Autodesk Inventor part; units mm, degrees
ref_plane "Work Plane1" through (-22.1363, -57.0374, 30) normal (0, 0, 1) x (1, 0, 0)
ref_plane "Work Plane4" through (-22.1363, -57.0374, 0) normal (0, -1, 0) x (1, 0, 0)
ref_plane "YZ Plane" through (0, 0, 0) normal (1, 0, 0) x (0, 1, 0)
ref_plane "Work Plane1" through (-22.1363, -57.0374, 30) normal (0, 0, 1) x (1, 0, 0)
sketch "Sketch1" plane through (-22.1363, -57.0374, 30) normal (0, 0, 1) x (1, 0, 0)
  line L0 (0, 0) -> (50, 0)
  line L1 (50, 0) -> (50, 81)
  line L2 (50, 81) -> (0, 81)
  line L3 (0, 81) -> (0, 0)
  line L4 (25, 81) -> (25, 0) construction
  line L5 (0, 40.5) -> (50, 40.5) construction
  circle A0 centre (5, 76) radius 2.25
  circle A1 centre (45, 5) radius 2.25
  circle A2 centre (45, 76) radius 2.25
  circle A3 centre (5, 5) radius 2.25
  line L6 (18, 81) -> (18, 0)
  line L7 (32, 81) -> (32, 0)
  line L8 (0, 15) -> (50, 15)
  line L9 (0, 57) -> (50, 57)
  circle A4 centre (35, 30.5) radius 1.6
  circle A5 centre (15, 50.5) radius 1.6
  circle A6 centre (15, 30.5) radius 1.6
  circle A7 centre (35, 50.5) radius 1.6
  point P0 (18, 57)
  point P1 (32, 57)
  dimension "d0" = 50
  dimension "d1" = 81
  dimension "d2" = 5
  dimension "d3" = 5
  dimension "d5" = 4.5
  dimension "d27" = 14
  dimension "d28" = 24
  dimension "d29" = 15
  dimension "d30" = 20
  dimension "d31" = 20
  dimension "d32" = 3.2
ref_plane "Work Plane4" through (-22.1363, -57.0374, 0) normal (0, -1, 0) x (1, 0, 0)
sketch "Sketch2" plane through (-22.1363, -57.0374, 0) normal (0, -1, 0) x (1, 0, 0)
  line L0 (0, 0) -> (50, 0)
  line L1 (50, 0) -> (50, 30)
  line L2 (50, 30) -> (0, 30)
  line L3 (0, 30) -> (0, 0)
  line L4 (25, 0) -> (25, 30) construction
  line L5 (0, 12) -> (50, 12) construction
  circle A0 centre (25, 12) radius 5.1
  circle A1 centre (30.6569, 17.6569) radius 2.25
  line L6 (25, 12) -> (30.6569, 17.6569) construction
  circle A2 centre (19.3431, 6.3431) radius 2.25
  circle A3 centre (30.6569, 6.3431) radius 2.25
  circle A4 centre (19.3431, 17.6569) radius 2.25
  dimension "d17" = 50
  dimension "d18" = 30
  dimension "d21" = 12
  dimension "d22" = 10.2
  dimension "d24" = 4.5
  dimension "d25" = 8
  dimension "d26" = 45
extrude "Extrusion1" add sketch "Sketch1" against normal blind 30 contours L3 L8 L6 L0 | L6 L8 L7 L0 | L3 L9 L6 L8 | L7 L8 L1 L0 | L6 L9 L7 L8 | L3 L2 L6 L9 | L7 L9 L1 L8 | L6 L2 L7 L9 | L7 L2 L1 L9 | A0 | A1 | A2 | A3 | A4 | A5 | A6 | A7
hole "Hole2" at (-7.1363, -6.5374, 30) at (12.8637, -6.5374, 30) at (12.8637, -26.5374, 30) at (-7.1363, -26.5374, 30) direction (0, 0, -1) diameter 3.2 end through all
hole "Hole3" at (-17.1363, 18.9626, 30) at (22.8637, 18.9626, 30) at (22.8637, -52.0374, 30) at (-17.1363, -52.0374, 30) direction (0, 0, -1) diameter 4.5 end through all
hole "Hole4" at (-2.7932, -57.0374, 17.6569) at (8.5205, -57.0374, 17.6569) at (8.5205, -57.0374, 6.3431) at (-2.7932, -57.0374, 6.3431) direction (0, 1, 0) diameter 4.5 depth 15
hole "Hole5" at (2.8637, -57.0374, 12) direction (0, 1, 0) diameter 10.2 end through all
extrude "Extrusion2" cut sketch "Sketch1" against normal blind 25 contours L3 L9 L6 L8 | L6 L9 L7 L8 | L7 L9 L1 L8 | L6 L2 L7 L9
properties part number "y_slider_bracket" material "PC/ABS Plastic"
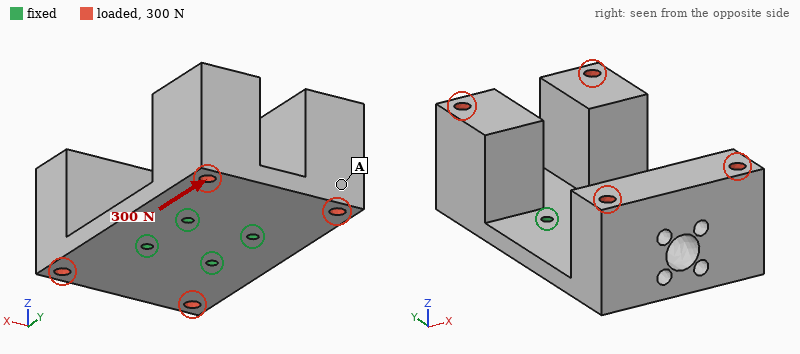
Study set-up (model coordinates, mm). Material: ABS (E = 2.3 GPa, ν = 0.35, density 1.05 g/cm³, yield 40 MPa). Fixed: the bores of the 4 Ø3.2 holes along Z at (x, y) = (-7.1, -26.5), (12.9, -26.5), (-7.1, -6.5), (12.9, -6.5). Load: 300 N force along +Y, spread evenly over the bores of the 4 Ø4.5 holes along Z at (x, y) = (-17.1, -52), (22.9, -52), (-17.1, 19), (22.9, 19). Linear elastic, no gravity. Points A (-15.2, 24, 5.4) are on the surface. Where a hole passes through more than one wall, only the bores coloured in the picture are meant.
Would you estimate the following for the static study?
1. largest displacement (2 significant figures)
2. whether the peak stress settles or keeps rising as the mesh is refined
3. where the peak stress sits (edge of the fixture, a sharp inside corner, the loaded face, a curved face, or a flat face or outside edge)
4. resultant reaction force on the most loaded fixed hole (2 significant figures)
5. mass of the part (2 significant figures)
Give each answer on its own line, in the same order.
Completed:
1.0 mm
keeps rising
edge of the fixture
86 N
59 g
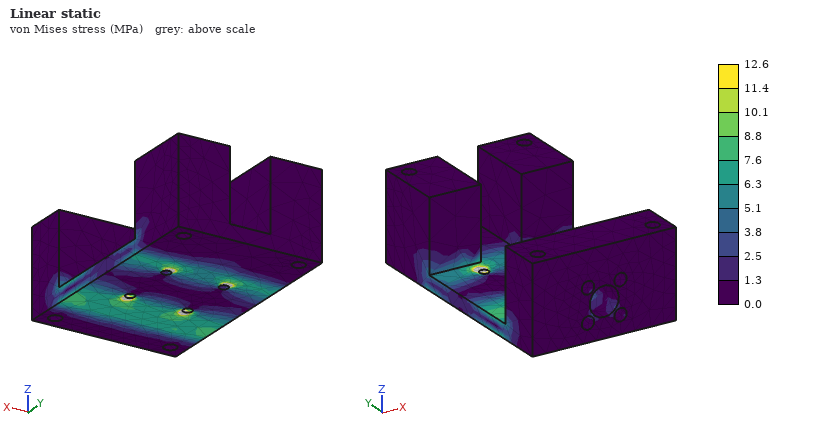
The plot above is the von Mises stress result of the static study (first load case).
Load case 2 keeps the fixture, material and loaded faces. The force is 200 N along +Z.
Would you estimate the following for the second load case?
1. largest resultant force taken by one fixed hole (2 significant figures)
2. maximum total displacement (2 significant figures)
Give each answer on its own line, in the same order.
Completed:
51 N
0.99 mm
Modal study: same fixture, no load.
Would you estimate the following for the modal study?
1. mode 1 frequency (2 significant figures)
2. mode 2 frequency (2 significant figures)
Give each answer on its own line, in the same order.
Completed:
400 Hz
470 Hz
